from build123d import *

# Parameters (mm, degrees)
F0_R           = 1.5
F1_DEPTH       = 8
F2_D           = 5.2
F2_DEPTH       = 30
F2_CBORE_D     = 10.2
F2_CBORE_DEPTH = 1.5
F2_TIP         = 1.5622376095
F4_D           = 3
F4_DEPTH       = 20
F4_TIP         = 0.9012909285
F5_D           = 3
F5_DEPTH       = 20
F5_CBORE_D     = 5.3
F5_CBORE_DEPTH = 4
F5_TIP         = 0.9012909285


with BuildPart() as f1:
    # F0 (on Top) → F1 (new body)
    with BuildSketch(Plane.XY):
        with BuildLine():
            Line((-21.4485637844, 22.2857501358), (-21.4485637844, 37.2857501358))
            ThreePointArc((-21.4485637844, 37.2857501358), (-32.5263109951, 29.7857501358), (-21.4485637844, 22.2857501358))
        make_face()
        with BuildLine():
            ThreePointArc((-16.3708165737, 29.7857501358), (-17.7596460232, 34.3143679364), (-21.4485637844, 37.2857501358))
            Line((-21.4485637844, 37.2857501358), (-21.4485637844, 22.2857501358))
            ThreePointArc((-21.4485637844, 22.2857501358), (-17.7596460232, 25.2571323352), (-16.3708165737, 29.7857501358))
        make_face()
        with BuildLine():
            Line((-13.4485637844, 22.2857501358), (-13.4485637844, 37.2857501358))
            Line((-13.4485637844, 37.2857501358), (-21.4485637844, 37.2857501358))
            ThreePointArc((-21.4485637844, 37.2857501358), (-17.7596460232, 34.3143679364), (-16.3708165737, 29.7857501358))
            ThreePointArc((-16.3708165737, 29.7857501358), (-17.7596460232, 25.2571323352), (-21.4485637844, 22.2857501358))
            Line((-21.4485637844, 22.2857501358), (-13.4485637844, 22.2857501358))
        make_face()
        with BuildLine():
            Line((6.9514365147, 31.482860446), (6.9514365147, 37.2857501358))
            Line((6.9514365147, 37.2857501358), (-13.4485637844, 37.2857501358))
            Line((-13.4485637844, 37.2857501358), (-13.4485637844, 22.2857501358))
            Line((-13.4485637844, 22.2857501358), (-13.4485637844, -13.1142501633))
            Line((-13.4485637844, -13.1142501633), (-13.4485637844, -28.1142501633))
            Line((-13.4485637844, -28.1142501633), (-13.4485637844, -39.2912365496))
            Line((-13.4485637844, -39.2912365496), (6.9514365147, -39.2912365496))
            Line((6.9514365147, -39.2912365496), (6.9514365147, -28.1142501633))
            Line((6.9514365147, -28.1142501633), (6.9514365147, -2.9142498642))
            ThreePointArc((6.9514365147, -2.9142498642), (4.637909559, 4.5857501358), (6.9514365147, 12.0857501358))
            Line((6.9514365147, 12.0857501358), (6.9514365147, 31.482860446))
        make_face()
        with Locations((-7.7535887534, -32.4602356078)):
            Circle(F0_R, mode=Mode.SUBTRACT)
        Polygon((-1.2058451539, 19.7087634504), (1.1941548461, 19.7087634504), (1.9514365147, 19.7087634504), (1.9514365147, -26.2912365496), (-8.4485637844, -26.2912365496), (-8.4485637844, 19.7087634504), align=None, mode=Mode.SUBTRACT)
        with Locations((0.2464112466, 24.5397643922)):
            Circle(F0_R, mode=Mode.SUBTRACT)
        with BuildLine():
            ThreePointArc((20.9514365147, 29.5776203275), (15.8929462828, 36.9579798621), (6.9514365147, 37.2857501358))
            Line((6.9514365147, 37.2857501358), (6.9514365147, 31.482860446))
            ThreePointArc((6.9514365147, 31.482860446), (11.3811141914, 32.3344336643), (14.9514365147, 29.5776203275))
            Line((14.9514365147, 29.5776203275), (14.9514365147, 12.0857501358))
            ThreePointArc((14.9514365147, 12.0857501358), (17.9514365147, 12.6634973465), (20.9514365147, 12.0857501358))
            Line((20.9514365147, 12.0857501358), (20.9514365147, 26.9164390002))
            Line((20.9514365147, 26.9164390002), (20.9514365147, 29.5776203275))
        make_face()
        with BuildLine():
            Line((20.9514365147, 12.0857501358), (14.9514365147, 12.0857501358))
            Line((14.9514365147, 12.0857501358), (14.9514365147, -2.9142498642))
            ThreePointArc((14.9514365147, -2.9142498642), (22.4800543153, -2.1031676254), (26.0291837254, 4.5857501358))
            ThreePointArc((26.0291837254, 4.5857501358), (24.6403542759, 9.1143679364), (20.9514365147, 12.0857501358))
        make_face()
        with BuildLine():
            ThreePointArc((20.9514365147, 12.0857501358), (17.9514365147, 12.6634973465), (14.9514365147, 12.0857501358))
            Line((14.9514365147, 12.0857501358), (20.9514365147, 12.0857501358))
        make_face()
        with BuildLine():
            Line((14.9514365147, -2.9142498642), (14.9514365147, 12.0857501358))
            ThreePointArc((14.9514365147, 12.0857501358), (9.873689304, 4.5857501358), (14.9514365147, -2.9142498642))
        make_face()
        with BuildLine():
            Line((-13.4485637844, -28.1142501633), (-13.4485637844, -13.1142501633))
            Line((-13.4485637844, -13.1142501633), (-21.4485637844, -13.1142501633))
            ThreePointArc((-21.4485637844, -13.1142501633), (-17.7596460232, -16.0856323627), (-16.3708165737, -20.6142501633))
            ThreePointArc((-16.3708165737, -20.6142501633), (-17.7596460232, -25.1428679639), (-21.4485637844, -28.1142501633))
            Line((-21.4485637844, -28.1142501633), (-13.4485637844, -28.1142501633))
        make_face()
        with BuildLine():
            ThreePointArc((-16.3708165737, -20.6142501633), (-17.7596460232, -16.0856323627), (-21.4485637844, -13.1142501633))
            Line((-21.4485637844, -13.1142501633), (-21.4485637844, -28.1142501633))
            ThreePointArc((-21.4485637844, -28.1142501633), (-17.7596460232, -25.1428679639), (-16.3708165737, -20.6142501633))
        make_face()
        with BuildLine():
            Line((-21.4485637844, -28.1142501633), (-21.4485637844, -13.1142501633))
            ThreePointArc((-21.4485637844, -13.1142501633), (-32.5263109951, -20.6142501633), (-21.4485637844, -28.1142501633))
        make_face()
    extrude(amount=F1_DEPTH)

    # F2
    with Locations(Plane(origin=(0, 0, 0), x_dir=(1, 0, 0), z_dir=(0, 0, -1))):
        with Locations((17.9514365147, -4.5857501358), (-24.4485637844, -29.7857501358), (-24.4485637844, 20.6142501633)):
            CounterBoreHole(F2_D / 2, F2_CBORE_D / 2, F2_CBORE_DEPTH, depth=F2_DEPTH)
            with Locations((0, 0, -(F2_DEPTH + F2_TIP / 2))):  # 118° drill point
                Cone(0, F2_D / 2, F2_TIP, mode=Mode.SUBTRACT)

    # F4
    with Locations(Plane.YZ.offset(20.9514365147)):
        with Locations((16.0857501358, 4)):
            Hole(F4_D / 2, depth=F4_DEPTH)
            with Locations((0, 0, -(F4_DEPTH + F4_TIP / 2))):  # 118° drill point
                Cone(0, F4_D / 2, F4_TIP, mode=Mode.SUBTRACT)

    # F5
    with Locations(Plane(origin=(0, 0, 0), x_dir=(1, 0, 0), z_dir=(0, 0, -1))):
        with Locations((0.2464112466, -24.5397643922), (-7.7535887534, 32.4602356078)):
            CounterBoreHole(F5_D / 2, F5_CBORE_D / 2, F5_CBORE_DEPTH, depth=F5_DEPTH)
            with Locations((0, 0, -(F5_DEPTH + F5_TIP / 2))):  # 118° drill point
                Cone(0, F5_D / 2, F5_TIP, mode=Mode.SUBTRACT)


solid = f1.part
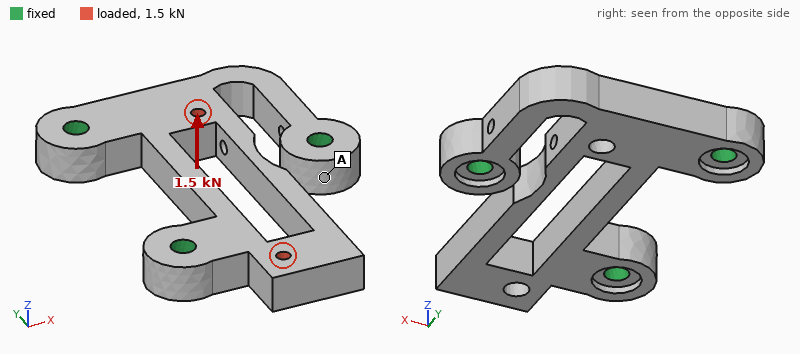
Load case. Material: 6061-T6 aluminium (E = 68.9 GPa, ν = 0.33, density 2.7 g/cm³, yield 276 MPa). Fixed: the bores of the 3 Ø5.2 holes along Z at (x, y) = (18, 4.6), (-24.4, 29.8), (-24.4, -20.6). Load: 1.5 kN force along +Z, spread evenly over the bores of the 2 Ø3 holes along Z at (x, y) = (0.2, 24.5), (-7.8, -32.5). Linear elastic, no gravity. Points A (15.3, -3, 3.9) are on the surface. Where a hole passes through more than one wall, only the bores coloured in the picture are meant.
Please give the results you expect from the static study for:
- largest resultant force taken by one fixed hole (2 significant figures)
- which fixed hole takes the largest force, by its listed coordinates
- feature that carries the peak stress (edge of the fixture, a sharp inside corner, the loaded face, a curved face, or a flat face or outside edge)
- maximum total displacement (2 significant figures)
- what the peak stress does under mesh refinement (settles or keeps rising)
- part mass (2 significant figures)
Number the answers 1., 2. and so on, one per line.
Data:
1. 860 N
2. (-24.4, -20.6)
3. edge of the fixture
4. 0.16 mm
5. keeps rising
6. 40 g
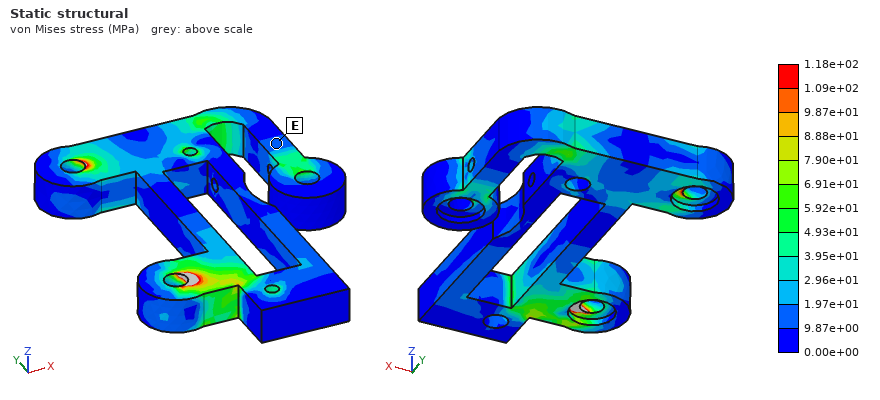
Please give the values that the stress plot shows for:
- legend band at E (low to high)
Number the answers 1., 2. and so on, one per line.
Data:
1. 9.87e+00 to 1.97e+01 MPa
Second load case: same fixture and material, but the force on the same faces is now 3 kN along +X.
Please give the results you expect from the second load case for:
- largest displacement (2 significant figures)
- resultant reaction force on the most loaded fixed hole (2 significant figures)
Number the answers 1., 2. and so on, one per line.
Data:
1. 66 µm
2. 1.6 kN
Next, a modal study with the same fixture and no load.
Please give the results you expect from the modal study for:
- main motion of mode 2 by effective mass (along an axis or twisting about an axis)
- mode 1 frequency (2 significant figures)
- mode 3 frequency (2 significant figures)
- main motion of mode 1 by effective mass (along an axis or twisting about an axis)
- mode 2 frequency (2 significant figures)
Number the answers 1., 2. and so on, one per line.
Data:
1. along Z
2. 4000 Hz
3. 7900 Hz
4. along Z
5. 5900 Hz
